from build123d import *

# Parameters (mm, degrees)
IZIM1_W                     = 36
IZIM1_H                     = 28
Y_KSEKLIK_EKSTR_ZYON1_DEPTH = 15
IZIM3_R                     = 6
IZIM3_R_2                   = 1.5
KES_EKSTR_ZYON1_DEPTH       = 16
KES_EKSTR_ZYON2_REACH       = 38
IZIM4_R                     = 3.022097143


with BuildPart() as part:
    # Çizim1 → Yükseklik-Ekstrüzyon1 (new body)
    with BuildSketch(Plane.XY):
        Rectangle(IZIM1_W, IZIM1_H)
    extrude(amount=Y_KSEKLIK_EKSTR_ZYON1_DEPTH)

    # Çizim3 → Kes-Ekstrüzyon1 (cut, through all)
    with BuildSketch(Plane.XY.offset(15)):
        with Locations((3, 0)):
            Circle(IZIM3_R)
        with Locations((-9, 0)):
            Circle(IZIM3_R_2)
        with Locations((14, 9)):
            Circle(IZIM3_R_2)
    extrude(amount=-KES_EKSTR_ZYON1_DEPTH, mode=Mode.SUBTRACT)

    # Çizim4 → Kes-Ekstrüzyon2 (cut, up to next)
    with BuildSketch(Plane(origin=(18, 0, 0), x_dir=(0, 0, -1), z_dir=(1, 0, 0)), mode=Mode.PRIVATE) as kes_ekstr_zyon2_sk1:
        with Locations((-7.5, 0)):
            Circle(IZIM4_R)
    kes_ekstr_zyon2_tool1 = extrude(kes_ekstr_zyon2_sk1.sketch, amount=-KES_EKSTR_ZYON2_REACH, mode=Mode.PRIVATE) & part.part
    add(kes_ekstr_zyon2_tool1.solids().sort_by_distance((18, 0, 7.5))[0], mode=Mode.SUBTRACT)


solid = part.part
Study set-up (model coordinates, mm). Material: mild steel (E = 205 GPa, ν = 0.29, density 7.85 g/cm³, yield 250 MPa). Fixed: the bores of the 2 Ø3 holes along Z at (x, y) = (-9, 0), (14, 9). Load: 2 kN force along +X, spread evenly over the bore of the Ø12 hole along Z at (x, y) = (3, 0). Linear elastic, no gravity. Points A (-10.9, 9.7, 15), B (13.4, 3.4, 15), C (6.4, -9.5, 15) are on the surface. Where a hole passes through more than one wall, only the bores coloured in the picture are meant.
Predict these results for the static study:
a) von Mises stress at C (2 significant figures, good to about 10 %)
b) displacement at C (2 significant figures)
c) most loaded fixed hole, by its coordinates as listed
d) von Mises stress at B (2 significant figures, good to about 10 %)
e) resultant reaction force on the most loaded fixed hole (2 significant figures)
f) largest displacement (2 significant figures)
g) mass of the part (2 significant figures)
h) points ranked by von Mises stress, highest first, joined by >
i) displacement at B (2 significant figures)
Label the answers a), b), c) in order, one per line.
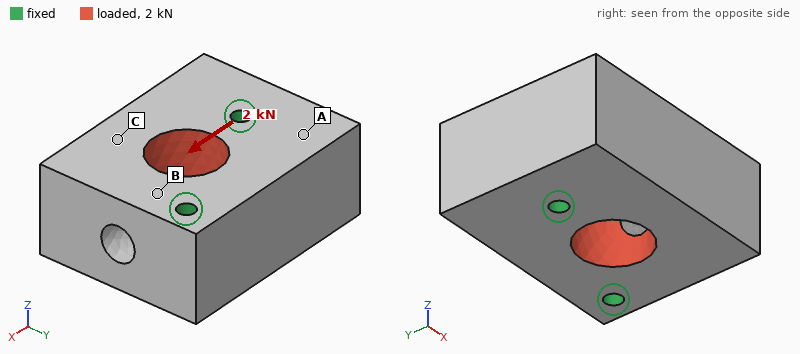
a) 3.6 MPa
b) 0.68 µm
c) (-9, 0)
d) 7.1 MPa
e) 1.3 kN
f) 0.87 µm
g) 100 g
h) B > C > A
i) 0.39 µm
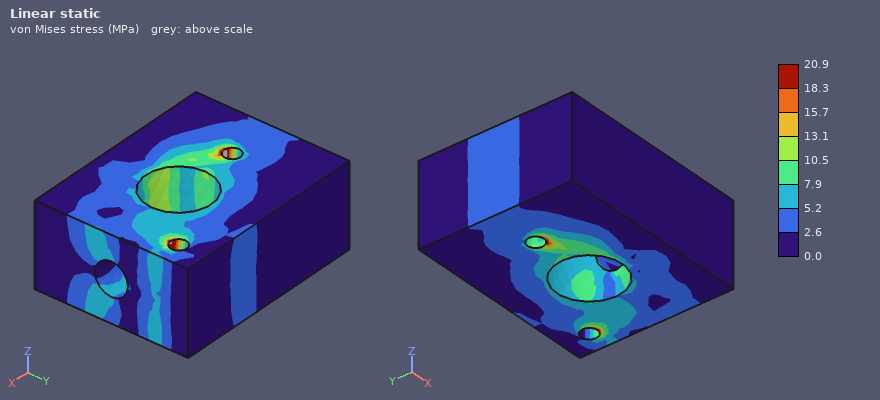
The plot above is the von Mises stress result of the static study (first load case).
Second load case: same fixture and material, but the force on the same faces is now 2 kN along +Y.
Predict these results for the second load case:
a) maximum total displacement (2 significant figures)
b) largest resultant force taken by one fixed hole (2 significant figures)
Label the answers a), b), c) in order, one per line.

a) 0.71 µm
b) 1.0 kN
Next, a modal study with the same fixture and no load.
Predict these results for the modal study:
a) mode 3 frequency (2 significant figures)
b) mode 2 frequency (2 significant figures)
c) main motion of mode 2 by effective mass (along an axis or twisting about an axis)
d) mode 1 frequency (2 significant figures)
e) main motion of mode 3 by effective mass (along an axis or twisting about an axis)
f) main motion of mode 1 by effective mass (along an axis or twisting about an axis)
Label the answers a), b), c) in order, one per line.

a) 32 kHz
b) 25 kHz
c) along X
d) 18 kHz
e) twisting about X
f) along Z
